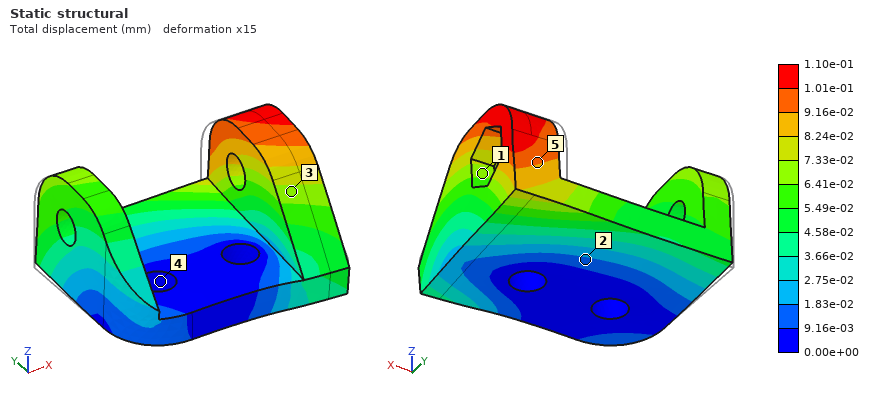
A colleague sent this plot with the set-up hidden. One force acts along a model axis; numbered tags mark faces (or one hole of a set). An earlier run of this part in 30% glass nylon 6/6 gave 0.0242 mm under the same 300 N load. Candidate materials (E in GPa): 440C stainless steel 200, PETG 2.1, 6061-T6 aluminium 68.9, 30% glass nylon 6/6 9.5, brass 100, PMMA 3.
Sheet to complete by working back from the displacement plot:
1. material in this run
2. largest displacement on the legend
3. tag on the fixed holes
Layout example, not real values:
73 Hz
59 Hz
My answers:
PETG
1.10e-01 mm
4
